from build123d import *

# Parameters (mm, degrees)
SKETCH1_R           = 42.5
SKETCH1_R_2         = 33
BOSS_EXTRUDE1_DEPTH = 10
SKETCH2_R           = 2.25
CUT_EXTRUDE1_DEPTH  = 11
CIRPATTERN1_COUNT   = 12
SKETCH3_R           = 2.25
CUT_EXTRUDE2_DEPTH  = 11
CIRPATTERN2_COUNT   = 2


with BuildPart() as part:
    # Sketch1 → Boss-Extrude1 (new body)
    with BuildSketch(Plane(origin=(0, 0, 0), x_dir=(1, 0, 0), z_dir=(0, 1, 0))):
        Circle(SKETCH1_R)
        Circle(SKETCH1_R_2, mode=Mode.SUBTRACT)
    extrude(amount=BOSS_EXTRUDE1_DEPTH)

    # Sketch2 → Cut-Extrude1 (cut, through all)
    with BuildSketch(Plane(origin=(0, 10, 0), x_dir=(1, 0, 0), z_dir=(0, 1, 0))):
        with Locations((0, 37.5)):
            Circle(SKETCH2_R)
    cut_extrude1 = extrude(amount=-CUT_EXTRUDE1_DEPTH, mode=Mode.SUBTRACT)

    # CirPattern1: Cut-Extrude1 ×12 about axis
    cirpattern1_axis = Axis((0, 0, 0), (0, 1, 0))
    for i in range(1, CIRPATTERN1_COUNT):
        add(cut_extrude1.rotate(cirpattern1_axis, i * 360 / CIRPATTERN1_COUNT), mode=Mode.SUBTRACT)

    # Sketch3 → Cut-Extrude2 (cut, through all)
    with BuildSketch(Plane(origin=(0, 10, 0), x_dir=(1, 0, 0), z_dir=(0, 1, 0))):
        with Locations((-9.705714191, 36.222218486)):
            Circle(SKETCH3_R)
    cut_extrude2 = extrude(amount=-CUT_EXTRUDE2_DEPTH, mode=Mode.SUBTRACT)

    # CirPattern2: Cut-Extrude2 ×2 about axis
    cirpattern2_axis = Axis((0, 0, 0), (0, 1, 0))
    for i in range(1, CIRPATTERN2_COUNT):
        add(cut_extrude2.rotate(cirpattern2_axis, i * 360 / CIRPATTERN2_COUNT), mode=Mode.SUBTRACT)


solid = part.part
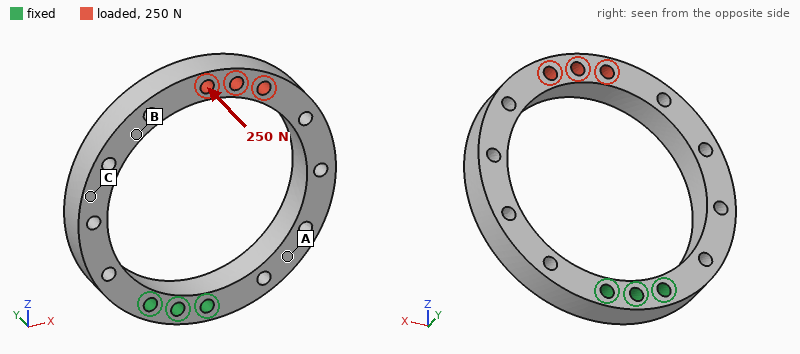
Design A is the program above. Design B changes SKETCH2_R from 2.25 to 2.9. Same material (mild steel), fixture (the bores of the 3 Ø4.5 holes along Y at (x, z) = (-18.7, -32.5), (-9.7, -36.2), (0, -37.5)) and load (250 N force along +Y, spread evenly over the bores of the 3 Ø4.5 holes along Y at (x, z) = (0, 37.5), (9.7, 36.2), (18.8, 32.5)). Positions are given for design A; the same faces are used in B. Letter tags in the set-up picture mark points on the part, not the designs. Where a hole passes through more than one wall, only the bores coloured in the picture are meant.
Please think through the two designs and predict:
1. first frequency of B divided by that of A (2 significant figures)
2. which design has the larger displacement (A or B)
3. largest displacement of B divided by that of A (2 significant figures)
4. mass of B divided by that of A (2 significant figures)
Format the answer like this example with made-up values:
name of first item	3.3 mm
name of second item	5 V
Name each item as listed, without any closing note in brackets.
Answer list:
first frequency of B divided by that of A	0.97
which design has the larger displacement	B
largest displacement of B divided by that of A	1.1
mass of B divided by that of A	0.94
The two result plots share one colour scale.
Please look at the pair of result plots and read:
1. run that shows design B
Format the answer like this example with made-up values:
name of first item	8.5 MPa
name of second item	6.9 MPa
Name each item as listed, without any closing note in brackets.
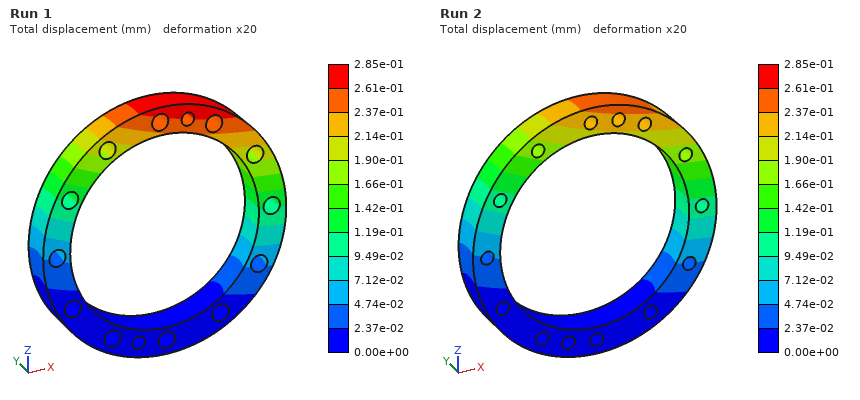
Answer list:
run that shows design B	Run 1
